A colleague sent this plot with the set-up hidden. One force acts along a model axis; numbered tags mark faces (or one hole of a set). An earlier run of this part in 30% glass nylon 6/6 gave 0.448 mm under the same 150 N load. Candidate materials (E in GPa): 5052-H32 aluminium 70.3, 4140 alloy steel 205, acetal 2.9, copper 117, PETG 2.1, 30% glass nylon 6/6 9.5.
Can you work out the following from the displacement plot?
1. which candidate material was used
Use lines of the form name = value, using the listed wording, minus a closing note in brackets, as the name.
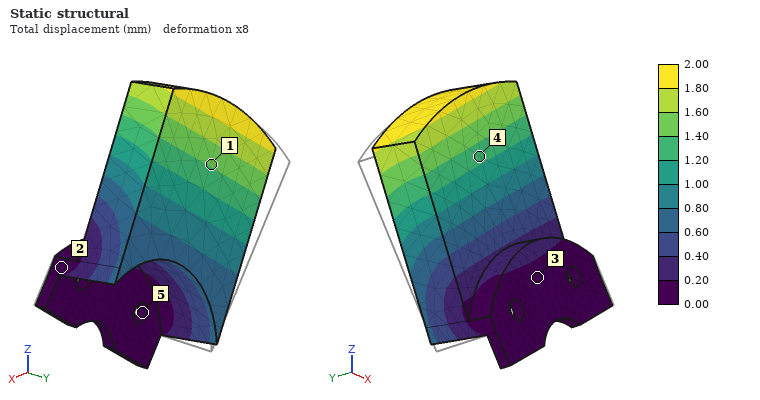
which candidate material was used = PETG
